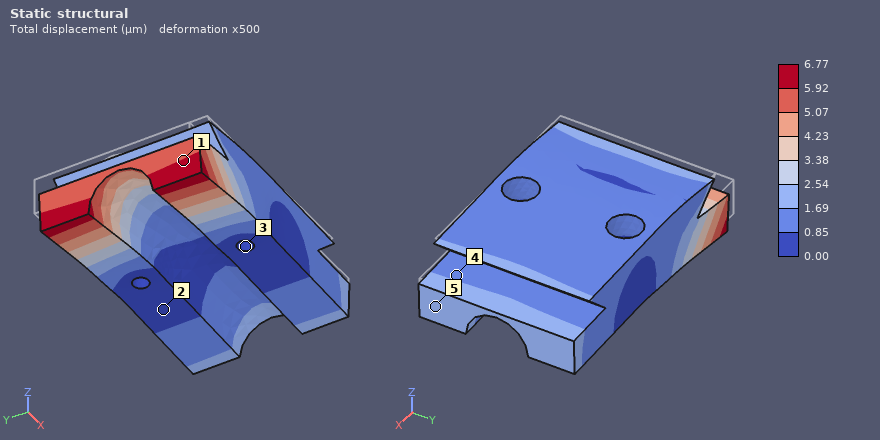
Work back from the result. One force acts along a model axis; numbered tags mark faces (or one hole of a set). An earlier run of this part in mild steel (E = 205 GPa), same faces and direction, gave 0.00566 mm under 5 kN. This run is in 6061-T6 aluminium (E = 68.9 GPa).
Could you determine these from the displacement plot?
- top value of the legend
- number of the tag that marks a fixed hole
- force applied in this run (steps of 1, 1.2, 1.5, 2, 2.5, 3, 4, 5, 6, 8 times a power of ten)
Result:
6.77 µm
3
2 kN
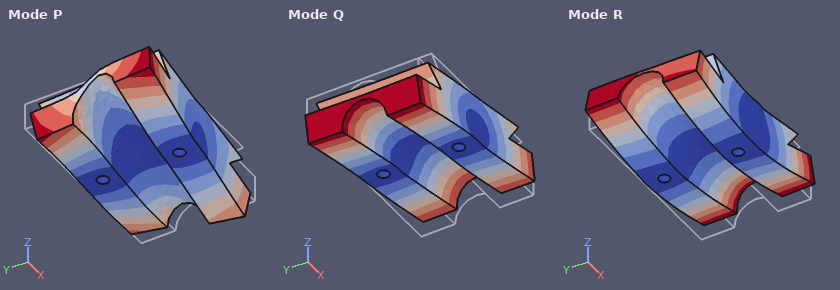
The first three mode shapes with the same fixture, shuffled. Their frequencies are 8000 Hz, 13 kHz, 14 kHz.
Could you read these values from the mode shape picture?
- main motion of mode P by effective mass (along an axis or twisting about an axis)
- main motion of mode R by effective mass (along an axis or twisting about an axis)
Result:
twisting about Z
along Z
